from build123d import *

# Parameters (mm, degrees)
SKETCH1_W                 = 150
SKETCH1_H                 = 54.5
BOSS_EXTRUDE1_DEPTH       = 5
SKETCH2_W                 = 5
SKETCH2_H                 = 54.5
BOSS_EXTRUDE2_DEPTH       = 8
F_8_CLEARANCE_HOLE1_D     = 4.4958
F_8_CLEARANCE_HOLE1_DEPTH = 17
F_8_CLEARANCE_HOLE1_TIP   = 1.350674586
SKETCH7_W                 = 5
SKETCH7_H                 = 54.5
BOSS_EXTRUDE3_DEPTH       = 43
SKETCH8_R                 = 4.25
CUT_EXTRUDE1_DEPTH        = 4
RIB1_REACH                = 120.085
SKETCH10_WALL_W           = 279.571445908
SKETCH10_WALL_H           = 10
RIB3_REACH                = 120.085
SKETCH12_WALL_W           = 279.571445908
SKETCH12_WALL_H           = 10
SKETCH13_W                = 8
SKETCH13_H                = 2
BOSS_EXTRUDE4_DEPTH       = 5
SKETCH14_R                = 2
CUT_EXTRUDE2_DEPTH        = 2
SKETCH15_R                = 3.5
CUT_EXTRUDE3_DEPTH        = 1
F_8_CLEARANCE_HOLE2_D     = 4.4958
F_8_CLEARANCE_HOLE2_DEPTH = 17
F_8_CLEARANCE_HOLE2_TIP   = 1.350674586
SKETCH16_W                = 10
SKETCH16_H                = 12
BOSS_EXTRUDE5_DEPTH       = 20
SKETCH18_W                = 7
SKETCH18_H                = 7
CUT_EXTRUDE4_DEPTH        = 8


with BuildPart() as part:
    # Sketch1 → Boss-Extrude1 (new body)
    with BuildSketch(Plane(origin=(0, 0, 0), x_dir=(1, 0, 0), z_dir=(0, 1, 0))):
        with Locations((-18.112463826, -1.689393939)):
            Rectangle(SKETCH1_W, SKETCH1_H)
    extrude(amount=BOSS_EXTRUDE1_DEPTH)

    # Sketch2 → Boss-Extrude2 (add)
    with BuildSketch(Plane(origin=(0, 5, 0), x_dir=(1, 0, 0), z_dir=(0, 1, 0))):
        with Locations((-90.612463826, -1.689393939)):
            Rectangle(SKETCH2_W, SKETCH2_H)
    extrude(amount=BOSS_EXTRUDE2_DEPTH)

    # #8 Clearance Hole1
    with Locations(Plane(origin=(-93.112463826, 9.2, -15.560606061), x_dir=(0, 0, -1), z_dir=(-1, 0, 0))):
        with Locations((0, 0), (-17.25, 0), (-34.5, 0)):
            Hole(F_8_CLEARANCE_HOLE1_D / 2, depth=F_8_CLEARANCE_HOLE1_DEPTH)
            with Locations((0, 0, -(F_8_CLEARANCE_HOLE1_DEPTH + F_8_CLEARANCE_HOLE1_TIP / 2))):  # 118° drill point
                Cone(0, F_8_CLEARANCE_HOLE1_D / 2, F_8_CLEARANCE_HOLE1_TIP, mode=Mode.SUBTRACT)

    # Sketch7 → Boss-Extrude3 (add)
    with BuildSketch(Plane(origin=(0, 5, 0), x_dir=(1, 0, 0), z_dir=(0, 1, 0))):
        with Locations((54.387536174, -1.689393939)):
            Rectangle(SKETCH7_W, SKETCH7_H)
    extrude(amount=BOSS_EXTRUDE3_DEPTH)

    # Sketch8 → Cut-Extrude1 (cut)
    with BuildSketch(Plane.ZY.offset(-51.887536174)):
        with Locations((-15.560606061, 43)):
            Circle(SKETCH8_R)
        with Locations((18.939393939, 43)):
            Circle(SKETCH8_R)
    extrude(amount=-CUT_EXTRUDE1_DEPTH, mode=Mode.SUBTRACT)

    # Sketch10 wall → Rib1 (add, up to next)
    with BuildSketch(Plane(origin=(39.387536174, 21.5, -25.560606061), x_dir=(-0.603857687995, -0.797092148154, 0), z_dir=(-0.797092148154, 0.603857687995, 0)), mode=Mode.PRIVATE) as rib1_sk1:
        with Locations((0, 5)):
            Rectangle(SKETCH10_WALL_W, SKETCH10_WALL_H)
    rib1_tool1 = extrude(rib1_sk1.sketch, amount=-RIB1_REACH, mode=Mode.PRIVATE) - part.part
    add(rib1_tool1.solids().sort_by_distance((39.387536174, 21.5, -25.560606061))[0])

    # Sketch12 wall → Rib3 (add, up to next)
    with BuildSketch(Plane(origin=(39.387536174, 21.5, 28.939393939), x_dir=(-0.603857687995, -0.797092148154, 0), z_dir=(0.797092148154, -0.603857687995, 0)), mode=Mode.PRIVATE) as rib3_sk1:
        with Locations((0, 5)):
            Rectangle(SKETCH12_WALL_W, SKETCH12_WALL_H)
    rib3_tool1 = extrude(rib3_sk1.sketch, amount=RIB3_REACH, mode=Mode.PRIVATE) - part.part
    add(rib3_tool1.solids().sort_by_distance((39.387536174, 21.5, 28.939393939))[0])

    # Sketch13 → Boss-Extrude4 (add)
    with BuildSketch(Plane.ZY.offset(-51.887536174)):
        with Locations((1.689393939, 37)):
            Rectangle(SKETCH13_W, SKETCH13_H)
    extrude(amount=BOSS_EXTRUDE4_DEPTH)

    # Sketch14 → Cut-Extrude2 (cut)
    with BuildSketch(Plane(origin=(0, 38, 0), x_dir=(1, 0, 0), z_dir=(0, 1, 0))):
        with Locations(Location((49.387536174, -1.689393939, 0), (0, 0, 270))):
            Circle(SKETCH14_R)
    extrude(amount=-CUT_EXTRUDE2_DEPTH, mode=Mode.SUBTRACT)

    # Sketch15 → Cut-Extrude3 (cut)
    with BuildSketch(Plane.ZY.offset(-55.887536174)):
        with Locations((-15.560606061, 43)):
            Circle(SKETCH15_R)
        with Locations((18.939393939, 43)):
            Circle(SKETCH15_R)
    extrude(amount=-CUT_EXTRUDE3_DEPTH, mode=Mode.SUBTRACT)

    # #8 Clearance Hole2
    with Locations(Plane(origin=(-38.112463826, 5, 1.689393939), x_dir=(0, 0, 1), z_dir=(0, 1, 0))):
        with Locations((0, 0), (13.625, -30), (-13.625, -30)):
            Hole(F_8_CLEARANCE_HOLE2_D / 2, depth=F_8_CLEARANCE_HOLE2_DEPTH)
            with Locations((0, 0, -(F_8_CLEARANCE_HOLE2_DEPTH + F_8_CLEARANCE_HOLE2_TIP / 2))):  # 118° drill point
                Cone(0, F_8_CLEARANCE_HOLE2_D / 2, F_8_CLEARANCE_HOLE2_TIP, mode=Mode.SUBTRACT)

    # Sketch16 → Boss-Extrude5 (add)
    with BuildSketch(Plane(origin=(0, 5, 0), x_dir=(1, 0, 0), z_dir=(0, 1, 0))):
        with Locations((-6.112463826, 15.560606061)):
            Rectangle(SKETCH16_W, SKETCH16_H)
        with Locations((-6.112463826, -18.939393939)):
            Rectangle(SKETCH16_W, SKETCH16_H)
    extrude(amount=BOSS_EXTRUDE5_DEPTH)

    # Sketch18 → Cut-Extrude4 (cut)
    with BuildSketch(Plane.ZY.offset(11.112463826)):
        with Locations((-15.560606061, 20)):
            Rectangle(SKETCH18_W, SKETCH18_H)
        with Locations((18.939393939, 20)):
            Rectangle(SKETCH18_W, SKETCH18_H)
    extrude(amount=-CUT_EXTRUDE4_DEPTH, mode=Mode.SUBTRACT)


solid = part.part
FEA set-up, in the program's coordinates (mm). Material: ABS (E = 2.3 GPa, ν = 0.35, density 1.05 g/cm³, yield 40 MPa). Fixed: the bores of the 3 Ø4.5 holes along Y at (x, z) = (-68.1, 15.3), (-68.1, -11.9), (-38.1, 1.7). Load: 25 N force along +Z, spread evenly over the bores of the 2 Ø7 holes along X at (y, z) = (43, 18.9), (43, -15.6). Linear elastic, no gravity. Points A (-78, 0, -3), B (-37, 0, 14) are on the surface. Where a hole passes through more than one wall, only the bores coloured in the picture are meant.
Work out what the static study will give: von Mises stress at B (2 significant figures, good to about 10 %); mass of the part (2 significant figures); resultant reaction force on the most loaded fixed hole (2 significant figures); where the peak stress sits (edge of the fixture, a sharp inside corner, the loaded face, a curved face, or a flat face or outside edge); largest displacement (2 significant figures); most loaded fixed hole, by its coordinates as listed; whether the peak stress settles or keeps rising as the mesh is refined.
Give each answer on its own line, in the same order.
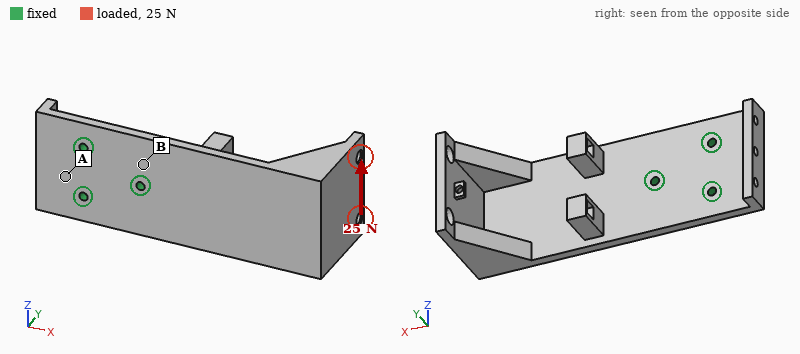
3.0 MPa
69 g
61 N
edge of the fixture
1.8 mm
(-38.1, 1.7)
keeps rising
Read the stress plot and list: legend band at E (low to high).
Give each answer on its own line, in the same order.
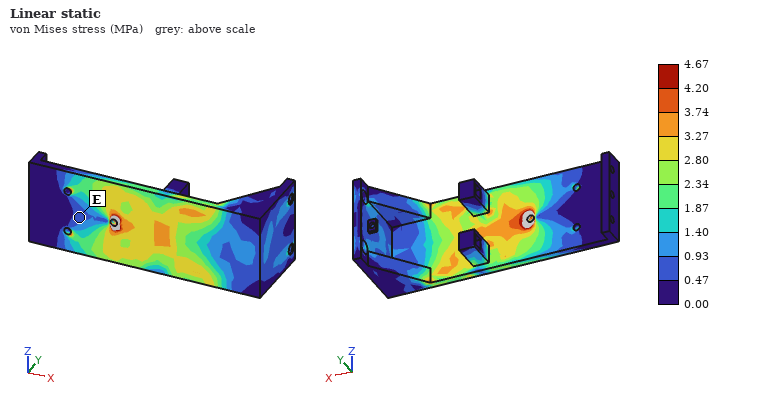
0.47 to 0.93 MPa
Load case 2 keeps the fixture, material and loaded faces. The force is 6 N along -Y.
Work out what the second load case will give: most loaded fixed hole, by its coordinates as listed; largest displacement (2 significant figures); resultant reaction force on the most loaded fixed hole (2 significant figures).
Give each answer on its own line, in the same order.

(-38.1, 1.7)
1.5 mm
18 N
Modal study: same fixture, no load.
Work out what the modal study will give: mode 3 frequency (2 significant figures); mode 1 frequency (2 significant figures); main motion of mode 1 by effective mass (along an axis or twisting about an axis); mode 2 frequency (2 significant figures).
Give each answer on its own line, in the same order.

410 Hz
68 Hz
along Y
190 Hz
